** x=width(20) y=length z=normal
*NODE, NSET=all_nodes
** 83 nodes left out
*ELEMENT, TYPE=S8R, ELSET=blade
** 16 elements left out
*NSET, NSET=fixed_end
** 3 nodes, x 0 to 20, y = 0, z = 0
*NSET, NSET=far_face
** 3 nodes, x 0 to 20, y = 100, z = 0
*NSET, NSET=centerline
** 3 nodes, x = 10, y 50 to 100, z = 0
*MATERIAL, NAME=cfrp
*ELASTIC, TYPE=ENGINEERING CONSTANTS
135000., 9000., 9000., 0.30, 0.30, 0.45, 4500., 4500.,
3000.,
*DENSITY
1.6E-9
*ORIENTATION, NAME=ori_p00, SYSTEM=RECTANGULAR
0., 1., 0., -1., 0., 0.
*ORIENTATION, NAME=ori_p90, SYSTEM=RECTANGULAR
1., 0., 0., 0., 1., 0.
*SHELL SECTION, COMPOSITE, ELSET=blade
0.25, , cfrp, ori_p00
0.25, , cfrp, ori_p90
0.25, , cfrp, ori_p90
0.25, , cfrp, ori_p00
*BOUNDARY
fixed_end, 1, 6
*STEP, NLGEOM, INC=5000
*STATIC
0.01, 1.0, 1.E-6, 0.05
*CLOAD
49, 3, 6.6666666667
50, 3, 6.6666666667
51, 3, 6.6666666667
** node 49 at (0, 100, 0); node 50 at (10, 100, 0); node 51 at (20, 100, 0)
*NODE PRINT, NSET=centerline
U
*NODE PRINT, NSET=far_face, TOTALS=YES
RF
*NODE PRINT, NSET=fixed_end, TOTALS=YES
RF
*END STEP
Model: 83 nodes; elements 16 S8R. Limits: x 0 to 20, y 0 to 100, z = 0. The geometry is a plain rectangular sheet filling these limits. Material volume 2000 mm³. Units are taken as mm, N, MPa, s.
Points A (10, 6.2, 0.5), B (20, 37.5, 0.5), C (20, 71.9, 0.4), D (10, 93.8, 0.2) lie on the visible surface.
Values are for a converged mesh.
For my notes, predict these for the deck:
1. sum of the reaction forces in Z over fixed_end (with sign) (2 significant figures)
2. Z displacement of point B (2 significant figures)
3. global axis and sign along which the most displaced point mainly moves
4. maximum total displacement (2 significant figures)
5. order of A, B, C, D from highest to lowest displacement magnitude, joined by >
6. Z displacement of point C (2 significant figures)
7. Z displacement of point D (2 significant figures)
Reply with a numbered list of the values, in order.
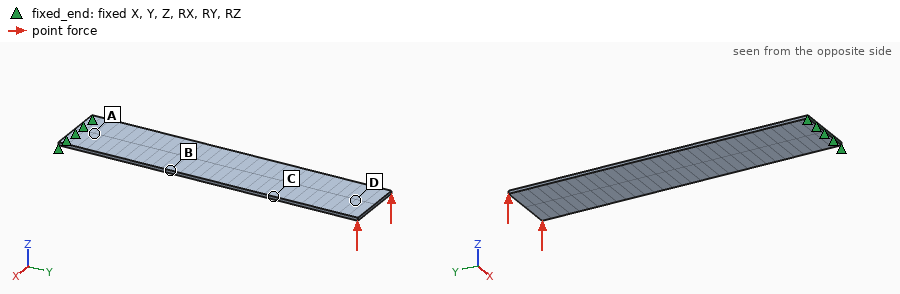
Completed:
1. -20 N
2. 5.7 mm
3. +Z
4. 31 mm
5. D > C > B > A
6. 18 mm
7. 27 mm
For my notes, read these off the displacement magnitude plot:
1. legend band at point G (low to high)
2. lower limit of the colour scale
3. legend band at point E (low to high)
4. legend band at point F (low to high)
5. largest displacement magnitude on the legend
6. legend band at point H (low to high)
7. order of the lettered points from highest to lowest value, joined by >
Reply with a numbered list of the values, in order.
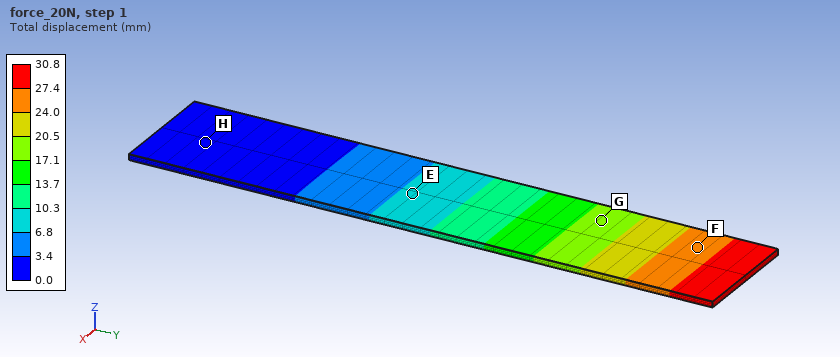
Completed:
1. 17.1 to 20.5 mm
2. 0.0 mm
3. 6.8 to 10.3 mm
4. 24.0 to 27.4 mm
5. 30.8 mm
6. 0.0 to 3.4 mm
7. F > G > E > H
